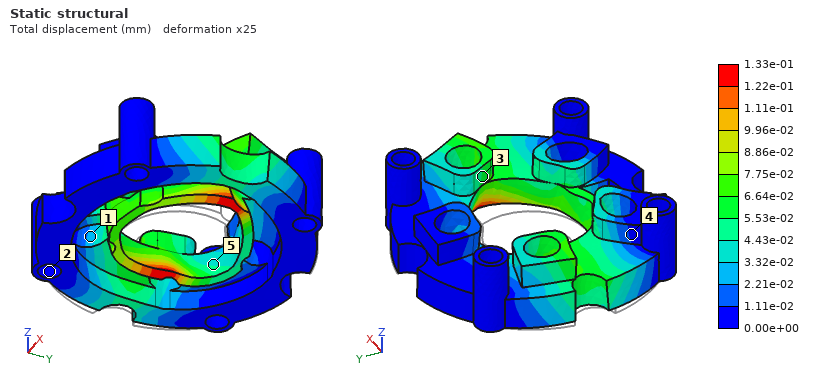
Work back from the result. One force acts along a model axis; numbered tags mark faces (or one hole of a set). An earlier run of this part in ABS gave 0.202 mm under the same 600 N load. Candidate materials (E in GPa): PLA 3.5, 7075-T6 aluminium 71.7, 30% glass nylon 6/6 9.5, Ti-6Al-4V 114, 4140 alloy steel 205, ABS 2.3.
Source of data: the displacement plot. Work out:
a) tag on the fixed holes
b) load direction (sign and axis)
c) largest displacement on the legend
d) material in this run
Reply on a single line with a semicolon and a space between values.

2; +X; 1.33e-01 mm; PLA
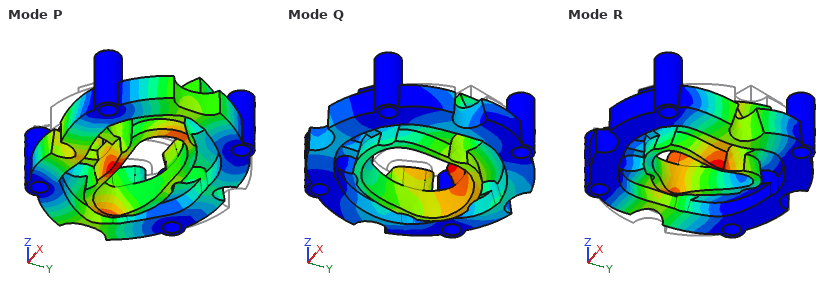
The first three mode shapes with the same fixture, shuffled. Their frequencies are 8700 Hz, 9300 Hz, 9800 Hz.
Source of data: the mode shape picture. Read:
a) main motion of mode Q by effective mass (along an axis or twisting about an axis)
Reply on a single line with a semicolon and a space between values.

along Z
